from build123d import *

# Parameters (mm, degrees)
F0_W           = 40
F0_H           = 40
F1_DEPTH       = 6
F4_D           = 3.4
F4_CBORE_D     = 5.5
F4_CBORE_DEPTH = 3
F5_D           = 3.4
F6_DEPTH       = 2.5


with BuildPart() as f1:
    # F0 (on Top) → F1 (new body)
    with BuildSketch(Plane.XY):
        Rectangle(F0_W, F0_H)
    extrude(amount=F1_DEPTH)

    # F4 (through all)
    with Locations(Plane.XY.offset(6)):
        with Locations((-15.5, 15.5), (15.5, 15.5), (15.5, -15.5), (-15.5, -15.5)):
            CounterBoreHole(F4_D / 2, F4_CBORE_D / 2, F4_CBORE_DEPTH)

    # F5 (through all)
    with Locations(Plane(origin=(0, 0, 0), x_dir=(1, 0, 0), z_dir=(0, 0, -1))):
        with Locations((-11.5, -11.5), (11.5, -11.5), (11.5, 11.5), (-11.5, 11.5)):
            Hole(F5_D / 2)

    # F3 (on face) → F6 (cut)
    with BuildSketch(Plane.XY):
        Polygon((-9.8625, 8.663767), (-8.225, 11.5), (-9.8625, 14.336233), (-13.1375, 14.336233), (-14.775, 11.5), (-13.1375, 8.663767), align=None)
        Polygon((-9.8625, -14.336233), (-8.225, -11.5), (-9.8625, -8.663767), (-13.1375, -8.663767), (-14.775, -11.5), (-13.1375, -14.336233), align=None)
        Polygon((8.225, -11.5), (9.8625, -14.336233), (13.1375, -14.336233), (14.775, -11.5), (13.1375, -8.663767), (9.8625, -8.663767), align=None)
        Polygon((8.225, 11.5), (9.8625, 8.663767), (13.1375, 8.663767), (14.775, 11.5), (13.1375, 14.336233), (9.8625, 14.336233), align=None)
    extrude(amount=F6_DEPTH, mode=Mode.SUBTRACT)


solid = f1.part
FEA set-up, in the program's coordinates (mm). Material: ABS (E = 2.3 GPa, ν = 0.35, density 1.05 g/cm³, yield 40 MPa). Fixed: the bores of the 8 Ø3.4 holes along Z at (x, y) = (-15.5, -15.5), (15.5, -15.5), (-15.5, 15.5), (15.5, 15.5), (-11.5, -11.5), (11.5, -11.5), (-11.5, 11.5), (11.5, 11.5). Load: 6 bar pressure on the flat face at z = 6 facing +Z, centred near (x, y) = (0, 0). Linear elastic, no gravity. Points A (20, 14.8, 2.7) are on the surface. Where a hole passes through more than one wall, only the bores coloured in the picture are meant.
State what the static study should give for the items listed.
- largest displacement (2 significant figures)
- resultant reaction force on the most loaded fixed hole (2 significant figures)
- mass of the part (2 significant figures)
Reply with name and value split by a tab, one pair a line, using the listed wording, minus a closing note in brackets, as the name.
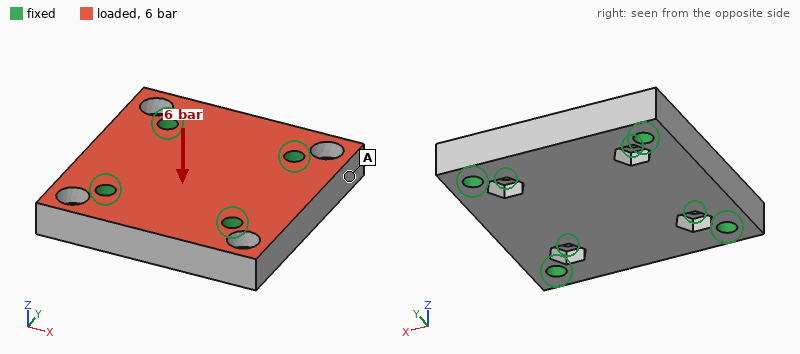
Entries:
largest displacement	44 µm
resultant reaction force on the most loaded fixed hole	180 N
mass of the part	9.2 g
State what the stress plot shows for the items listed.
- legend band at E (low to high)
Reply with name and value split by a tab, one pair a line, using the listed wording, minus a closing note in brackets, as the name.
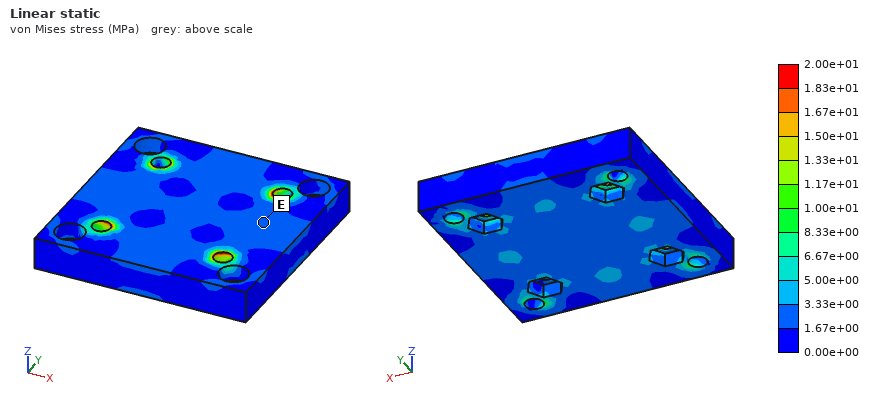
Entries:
legend band at E	1.67e+00 to 3.33e+00 MPa
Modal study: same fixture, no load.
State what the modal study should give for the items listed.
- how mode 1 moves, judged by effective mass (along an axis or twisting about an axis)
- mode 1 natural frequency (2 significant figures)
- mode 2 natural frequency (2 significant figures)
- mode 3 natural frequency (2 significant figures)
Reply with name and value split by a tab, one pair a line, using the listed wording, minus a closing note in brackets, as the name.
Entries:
how mode 1 moves, judged by effective mass	along Z
mode 1 natural frequency	8700 Hz
mode 2 natural frequency	9600 Hz
mode 3 natural frequency	9800 Hz
